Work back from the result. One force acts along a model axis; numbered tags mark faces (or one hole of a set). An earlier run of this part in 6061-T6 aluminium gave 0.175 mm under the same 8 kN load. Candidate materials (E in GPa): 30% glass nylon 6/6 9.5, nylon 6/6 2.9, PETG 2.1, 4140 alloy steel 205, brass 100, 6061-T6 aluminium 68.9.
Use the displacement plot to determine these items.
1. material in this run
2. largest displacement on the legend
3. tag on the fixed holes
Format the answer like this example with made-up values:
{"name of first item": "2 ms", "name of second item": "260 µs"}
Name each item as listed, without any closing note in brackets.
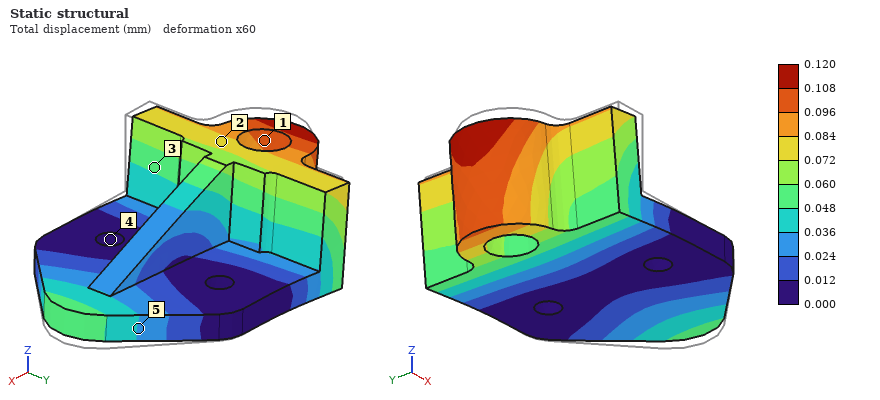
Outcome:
{"material in this run": "brass", "largest displacement on the legend": "0.120 mm", "tag on the fixed holes": "4"}
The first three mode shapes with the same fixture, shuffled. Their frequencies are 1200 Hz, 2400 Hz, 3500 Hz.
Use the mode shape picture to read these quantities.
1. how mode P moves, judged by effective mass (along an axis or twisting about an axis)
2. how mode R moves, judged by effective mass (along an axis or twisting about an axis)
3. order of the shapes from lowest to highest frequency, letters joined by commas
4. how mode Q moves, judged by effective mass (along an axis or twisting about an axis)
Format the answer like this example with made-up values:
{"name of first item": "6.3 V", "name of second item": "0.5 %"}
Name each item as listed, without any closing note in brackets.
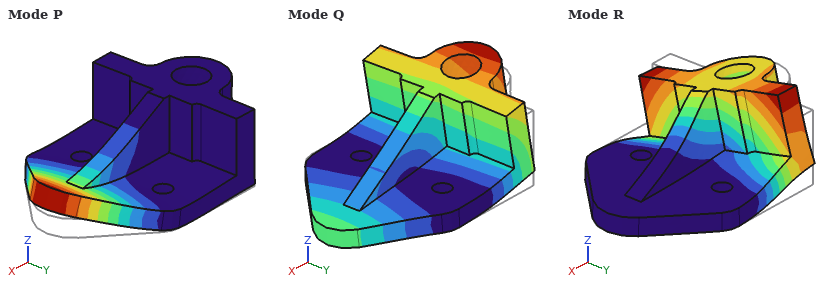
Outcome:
{"how mode P moves, judged by effective mass": "along Z", "how mode R moves, judged by effective mass": "along Y", "order of the shapes from lowest to highest frequency, letters joined by commas": "Q, R, P", "how mode Q moves, judged by effective mass": "along Z"}
